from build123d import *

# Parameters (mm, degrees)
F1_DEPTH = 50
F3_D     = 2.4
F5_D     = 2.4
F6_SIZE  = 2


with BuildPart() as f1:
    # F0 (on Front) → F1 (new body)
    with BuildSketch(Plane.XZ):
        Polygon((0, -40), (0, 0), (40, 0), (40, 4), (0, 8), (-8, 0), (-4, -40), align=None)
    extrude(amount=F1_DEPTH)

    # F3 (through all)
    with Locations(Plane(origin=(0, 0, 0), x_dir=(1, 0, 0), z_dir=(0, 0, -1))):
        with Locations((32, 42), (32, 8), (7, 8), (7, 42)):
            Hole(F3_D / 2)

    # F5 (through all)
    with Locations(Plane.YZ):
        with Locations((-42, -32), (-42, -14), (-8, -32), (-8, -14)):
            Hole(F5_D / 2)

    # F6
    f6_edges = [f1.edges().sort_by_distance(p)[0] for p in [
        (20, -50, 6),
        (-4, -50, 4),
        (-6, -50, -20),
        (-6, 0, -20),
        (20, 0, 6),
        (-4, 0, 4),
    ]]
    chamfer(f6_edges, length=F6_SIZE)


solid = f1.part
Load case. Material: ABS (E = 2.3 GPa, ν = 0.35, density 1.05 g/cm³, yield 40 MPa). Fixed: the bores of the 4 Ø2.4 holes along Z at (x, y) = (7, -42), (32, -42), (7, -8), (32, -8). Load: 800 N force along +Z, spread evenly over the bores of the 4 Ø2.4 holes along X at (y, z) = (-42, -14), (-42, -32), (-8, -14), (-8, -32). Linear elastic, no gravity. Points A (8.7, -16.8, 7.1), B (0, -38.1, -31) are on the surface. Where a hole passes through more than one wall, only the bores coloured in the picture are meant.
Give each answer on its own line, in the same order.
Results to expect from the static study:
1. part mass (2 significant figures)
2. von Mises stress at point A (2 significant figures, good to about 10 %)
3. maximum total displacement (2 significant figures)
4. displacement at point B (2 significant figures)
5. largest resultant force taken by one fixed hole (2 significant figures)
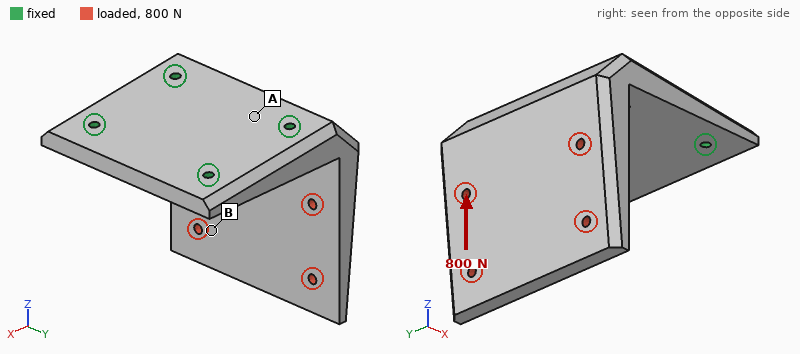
26 g
7.0 MPa
0.75 mm
0.60 mm
450 N
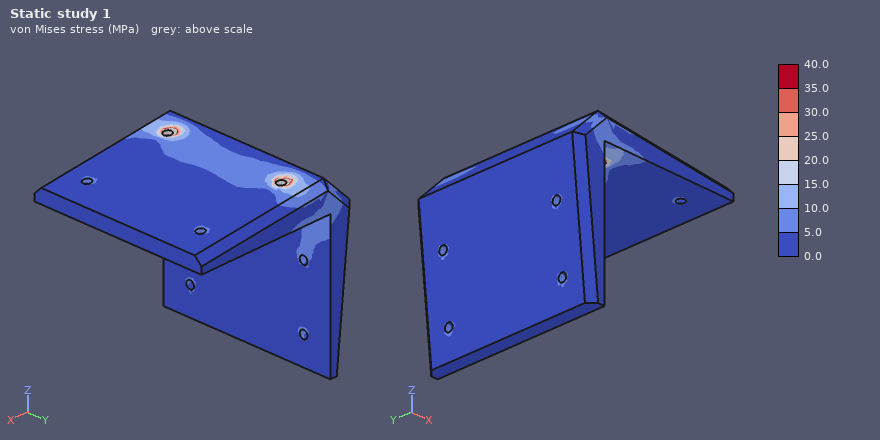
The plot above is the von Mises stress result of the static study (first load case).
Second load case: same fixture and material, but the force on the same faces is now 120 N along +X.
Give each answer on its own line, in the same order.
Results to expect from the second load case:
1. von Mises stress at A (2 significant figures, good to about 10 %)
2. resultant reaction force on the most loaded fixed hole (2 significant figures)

3.4 MPa
51 N
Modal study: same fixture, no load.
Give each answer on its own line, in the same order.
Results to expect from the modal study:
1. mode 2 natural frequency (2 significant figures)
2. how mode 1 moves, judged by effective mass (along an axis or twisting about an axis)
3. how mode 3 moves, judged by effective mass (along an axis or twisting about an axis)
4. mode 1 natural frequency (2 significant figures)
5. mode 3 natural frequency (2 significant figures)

1600 Hz
along X
along Y
730 Hz
2200 Hz
